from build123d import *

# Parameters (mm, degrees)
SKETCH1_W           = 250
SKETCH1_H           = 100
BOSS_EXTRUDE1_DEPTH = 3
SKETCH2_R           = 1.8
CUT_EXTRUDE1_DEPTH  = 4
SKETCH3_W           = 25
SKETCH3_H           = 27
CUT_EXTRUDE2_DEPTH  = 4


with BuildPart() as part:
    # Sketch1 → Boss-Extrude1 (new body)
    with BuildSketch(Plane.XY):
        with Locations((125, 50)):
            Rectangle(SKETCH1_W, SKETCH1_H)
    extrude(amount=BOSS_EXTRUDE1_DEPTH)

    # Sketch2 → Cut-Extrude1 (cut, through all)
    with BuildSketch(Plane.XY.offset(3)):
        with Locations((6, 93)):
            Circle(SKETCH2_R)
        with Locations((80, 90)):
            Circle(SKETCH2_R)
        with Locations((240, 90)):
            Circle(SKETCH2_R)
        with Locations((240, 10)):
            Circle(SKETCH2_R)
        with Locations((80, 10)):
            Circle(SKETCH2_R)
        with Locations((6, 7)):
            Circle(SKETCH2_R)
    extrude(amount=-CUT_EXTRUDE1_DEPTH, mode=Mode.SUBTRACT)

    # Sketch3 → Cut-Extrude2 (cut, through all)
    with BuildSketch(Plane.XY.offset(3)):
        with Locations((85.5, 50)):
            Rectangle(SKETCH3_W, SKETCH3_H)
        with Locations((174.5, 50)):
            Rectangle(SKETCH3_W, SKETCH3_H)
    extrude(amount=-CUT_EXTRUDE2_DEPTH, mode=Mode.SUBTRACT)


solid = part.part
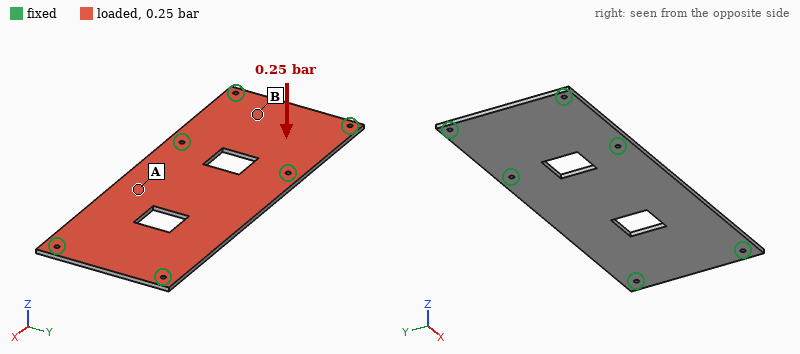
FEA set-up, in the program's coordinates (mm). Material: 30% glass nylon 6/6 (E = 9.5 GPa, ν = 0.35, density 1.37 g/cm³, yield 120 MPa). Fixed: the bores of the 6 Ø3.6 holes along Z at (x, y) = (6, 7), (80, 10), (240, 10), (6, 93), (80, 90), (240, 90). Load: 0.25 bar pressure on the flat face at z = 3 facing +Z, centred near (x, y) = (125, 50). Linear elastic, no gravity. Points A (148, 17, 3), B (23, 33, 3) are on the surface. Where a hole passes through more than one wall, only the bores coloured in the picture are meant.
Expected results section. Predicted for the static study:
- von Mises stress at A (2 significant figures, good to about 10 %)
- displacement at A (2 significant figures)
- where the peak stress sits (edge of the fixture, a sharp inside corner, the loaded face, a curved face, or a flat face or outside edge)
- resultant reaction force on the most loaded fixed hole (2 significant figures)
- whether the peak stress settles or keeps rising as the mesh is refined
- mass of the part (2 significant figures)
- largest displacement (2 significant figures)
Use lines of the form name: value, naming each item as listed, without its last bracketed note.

von Mises stress at A: 18 MPa
displacement at A: 2.5 mm
where the peak stress sits: edge of the fixture
resultant reaction force on the most loaded fixed hole: 140 N
whether the peak stress settles or keeps rising as the mesh is refined: keeps rising
mass of the part: 97 g
largest displacement: 2.8 mm
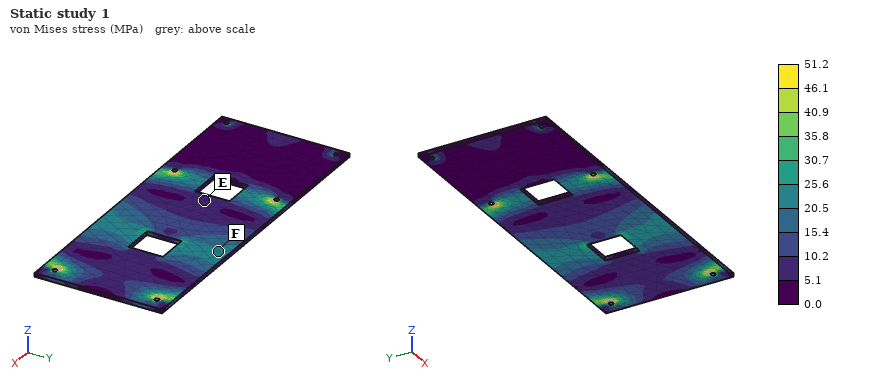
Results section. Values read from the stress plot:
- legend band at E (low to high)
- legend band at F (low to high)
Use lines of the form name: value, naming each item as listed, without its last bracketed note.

legend band at E: 5.1 to 10.2 MPa
legend band at F: 20.5 to 25.6 MPa
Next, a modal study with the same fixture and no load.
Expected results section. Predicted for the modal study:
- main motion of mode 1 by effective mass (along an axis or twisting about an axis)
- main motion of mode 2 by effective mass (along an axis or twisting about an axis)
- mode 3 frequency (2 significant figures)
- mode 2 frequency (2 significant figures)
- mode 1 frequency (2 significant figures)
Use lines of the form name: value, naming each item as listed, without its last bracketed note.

main motion of mode 1 by effective mass: along Z
main motion of mode 2 by effective mass: twisting about X
mode 3 frequency: 750 Hz
mode 2 frequency: 450 Hz
mode 1 frequency: 270 Hz
